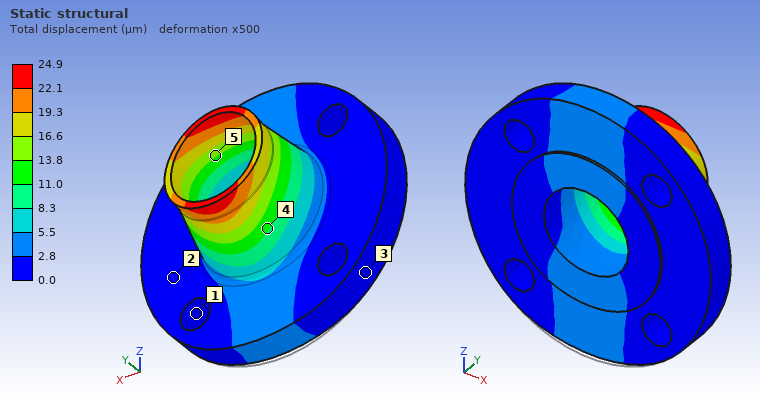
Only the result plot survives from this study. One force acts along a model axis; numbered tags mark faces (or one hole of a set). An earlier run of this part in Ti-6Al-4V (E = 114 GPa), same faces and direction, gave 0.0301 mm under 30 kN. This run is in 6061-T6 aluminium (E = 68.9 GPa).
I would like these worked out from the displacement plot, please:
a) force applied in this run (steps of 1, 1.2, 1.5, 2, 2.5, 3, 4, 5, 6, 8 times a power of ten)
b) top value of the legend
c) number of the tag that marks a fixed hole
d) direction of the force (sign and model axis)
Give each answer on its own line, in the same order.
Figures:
15 kN
24.9 µm
1
+Z
